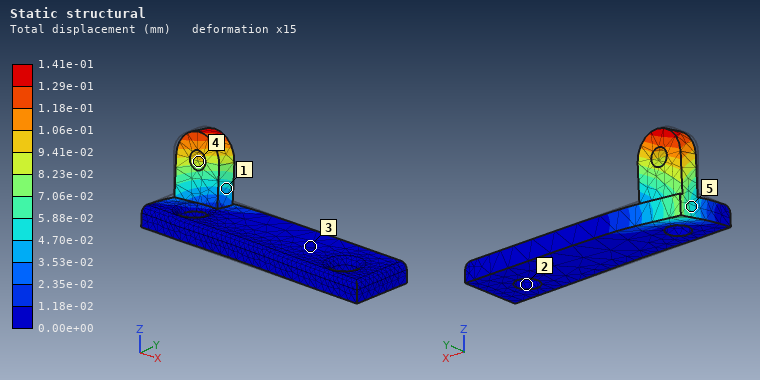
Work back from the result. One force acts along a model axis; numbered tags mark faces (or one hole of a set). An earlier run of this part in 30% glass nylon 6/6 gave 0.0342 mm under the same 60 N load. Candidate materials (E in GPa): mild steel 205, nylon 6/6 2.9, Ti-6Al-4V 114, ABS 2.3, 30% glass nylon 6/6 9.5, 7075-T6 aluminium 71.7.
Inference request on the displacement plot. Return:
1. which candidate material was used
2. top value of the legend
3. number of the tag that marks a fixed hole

ABS
1.41e-01 mm
2
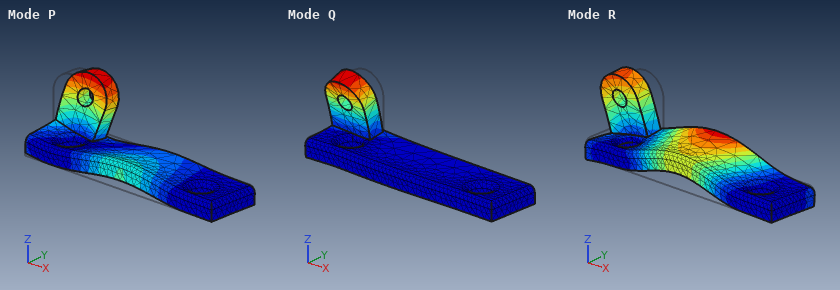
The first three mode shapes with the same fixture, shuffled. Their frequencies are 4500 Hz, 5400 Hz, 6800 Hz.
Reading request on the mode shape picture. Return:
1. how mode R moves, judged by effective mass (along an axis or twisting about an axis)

along Z
